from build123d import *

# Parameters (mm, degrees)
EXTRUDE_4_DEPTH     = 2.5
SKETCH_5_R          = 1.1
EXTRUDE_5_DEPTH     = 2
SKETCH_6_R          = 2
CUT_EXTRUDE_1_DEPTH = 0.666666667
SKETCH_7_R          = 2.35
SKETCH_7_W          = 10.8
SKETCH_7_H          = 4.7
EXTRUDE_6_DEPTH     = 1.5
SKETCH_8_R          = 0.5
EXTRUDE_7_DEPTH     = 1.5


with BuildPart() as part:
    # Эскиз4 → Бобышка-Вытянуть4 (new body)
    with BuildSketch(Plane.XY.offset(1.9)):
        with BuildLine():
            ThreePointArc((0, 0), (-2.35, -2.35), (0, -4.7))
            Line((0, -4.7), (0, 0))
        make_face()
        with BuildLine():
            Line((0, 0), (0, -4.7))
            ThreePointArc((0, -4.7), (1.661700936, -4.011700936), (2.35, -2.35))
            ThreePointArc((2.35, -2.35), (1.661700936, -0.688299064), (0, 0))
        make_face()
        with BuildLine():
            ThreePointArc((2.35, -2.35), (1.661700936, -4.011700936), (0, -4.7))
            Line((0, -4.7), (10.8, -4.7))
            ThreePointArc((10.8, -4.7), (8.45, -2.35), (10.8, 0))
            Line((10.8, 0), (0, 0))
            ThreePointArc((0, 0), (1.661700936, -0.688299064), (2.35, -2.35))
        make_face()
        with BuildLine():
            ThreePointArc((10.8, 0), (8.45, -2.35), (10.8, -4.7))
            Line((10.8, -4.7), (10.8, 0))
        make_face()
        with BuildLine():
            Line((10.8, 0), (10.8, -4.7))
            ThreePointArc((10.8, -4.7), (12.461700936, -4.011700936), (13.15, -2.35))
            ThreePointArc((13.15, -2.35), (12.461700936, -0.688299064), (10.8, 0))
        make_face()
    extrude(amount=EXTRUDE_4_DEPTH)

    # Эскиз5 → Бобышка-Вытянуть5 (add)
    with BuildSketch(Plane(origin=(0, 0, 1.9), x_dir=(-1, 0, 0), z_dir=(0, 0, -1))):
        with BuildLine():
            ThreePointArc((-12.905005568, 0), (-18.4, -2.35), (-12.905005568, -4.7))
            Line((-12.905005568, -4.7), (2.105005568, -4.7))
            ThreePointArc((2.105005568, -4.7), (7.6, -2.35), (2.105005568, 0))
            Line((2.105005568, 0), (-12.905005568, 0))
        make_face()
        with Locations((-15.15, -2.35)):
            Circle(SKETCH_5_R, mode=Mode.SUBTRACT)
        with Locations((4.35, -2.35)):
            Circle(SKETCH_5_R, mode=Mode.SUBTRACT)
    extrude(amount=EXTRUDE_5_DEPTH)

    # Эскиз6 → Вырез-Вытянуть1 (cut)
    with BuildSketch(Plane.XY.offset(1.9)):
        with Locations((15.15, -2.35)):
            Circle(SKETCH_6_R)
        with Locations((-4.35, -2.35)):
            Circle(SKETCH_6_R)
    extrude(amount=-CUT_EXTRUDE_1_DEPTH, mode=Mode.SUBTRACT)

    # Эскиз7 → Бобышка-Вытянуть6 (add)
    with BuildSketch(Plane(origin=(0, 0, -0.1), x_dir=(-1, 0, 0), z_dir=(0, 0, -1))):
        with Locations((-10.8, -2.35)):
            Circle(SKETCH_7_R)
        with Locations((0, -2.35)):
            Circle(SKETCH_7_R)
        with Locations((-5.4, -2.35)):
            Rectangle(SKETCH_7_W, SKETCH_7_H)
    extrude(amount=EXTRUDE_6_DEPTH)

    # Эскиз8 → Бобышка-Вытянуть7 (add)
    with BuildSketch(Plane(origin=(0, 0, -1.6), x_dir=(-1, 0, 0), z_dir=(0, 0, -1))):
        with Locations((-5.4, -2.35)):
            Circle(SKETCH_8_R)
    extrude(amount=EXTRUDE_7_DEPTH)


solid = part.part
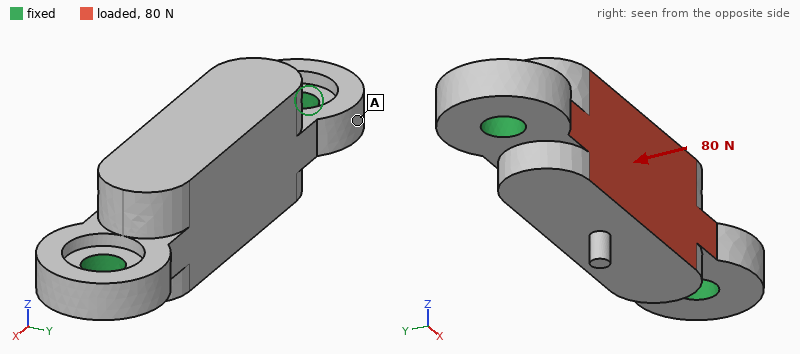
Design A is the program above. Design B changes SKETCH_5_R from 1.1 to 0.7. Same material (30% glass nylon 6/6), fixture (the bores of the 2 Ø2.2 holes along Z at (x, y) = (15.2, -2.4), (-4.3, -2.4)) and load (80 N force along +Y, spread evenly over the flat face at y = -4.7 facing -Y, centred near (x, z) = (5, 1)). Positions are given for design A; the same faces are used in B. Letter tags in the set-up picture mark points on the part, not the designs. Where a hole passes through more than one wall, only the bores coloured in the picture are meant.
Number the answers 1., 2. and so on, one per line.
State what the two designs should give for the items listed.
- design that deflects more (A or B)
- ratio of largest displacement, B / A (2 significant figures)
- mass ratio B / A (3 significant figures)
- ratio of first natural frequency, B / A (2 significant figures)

1. B
2. 1.5
3. 1.01
4. 0.82
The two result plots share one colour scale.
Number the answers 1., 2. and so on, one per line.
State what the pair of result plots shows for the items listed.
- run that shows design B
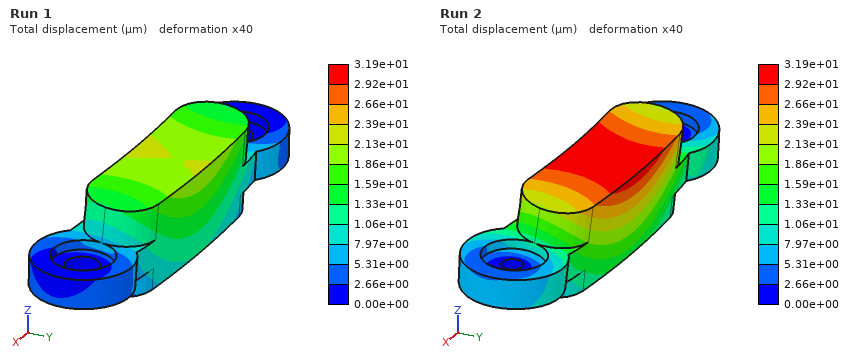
1. Run 2
